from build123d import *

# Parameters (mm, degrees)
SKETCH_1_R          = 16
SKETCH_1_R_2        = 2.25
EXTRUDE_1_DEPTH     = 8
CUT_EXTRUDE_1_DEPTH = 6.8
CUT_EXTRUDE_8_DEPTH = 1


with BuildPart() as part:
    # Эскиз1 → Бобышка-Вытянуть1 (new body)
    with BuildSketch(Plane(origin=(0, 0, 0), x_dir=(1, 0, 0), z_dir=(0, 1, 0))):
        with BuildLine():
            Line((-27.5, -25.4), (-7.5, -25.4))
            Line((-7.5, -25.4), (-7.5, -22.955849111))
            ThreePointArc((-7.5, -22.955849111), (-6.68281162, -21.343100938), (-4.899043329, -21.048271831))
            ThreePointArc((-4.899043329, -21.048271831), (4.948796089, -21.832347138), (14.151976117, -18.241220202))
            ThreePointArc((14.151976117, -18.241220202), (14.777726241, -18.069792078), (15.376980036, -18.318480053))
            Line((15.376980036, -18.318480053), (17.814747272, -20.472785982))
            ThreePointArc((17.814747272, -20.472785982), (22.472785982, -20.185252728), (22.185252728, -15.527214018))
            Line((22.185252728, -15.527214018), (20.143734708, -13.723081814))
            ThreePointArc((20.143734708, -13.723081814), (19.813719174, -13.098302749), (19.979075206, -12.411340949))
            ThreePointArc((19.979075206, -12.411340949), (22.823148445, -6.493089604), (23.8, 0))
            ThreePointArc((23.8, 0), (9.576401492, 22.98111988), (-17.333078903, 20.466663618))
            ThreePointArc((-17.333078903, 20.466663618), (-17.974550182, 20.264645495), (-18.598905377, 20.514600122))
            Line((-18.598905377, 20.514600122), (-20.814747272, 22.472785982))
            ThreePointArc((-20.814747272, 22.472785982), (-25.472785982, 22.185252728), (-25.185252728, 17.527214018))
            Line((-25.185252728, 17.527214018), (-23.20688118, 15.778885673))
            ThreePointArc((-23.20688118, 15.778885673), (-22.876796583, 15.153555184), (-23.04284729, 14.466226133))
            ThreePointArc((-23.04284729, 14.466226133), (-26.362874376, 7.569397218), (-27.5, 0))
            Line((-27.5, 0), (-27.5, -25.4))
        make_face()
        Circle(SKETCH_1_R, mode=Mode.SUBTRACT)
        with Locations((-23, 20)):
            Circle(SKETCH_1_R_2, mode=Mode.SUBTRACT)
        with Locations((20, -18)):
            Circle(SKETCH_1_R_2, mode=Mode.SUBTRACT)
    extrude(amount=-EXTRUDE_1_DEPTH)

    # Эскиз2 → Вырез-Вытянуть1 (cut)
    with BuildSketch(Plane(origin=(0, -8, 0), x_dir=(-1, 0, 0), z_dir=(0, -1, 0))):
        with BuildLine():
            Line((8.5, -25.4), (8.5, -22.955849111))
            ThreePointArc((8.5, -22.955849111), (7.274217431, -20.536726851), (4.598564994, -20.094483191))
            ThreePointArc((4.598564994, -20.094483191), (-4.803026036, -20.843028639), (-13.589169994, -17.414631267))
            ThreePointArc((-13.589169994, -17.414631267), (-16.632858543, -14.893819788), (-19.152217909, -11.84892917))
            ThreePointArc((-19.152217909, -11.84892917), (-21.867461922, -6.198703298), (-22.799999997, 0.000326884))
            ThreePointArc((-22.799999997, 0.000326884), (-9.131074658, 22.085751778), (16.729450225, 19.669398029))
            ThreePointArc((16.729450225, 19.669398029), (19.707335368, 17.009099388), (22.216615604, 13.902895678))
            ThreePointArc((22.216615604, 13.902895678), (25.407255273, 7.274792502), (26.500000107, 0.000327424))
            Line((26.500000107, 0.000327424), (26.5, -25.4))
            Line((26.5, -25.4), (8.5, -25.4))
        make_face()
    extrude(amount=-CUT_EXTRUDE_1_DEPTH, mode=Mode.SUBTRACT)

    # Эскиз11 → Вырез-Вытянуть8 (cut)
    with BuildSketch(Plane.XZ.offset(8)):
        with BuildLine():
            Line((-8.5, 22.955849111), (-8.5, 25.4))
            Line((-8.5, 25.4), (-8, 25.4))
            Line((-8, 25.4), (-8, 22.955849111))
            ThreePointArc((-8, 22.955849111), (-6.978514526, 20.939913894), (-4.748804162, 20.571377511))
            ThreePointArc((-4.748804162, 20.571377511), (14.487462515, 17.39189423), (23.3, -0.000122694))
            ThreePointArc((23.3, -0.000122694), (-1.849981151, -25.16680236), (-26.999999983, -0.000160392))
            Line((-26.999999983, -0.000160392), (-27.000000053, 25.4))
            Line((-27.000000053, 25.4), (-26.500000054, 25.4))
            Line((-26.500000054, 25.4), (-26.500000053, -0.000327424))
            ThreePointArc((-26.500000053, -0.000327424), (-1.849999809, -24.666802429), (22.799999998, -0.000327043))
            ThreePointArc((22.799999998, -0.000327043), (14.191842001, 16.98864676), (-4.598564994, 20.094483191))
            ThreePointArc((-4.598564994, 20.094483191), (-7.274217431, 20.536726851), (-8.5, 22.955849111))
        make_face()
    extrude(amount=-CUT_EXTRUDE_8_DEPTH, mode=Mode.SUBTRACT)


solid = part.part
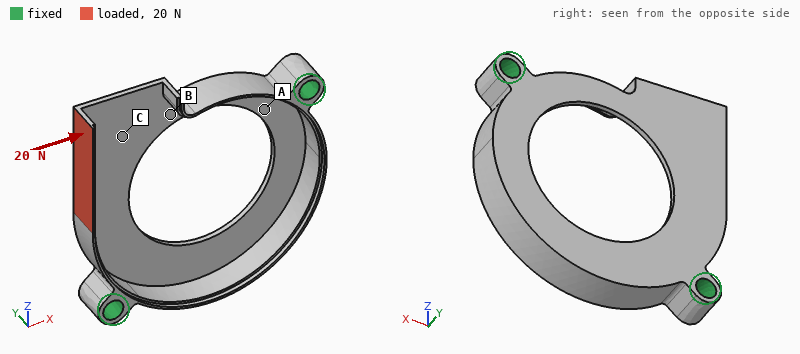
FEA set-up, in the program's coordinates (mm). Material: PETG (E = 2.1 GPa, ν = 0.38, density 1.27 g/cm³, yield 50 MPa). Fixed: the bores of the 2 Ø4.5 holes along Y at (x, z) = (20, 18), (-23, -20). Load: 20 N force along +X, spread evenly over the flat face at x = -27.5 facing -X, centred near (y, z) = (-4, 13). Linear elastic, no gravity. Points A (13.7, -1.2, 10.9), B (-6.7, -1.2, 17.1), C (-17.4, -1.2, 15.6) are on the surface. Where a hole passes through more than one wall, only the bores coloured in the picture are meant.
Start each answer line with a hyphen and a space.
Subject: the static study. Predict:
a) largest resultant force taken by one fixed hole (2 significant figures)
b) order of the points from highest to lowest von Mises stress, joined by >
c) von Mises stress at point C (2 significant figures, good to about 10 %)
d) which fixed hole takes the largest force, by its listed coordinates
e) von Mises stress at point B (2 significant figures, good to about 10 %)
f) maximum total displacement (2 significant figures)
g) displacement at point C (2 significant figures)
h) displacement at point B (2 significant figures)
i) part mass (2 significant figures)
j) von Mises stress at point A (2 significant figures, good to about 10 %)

- 15 N
- C > B > A
- 5.6 MPa
- (20, 18)
- 3.4 MPa
- 0.74 mm
- 0.24 mm
- 0.25 mm
- 3.7 g
- 1.5 MPa
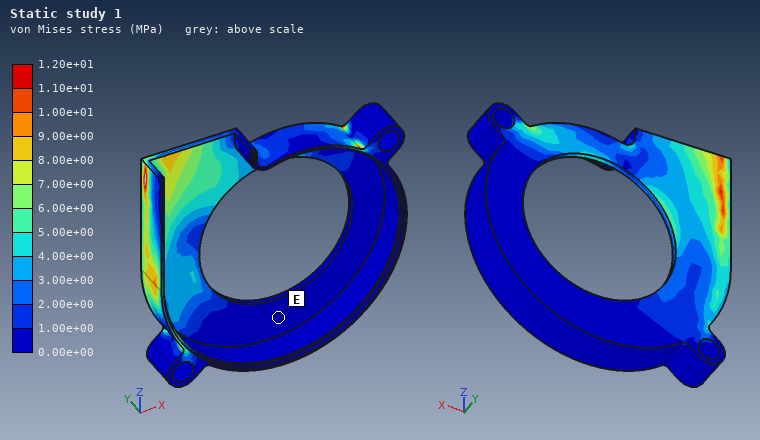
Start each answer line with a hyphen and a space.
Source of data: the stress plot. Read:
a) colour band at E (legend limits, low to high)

- 0.00e+00 to 1.00e+00 MPa
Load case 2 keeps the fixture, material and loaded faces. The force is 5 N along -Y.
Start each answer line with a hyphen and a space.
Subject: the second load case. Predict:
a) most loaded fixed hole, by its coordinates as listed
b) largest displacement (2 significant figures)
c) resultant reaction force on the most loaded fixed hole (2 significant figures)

- (-23, -20)
- 0.76 mm
- 4.9 N
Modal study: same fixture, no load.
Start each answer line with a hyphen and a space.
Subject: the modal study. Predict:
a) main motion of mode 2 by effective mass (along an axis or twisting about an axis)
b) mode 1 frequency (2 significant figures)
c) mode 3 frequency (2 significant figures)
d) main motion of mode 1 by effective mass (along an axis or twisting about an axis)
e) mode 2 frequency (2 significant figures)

- along Y
- 620 Hz
- 1200 Hz
- along Y
- 1000 Hz
